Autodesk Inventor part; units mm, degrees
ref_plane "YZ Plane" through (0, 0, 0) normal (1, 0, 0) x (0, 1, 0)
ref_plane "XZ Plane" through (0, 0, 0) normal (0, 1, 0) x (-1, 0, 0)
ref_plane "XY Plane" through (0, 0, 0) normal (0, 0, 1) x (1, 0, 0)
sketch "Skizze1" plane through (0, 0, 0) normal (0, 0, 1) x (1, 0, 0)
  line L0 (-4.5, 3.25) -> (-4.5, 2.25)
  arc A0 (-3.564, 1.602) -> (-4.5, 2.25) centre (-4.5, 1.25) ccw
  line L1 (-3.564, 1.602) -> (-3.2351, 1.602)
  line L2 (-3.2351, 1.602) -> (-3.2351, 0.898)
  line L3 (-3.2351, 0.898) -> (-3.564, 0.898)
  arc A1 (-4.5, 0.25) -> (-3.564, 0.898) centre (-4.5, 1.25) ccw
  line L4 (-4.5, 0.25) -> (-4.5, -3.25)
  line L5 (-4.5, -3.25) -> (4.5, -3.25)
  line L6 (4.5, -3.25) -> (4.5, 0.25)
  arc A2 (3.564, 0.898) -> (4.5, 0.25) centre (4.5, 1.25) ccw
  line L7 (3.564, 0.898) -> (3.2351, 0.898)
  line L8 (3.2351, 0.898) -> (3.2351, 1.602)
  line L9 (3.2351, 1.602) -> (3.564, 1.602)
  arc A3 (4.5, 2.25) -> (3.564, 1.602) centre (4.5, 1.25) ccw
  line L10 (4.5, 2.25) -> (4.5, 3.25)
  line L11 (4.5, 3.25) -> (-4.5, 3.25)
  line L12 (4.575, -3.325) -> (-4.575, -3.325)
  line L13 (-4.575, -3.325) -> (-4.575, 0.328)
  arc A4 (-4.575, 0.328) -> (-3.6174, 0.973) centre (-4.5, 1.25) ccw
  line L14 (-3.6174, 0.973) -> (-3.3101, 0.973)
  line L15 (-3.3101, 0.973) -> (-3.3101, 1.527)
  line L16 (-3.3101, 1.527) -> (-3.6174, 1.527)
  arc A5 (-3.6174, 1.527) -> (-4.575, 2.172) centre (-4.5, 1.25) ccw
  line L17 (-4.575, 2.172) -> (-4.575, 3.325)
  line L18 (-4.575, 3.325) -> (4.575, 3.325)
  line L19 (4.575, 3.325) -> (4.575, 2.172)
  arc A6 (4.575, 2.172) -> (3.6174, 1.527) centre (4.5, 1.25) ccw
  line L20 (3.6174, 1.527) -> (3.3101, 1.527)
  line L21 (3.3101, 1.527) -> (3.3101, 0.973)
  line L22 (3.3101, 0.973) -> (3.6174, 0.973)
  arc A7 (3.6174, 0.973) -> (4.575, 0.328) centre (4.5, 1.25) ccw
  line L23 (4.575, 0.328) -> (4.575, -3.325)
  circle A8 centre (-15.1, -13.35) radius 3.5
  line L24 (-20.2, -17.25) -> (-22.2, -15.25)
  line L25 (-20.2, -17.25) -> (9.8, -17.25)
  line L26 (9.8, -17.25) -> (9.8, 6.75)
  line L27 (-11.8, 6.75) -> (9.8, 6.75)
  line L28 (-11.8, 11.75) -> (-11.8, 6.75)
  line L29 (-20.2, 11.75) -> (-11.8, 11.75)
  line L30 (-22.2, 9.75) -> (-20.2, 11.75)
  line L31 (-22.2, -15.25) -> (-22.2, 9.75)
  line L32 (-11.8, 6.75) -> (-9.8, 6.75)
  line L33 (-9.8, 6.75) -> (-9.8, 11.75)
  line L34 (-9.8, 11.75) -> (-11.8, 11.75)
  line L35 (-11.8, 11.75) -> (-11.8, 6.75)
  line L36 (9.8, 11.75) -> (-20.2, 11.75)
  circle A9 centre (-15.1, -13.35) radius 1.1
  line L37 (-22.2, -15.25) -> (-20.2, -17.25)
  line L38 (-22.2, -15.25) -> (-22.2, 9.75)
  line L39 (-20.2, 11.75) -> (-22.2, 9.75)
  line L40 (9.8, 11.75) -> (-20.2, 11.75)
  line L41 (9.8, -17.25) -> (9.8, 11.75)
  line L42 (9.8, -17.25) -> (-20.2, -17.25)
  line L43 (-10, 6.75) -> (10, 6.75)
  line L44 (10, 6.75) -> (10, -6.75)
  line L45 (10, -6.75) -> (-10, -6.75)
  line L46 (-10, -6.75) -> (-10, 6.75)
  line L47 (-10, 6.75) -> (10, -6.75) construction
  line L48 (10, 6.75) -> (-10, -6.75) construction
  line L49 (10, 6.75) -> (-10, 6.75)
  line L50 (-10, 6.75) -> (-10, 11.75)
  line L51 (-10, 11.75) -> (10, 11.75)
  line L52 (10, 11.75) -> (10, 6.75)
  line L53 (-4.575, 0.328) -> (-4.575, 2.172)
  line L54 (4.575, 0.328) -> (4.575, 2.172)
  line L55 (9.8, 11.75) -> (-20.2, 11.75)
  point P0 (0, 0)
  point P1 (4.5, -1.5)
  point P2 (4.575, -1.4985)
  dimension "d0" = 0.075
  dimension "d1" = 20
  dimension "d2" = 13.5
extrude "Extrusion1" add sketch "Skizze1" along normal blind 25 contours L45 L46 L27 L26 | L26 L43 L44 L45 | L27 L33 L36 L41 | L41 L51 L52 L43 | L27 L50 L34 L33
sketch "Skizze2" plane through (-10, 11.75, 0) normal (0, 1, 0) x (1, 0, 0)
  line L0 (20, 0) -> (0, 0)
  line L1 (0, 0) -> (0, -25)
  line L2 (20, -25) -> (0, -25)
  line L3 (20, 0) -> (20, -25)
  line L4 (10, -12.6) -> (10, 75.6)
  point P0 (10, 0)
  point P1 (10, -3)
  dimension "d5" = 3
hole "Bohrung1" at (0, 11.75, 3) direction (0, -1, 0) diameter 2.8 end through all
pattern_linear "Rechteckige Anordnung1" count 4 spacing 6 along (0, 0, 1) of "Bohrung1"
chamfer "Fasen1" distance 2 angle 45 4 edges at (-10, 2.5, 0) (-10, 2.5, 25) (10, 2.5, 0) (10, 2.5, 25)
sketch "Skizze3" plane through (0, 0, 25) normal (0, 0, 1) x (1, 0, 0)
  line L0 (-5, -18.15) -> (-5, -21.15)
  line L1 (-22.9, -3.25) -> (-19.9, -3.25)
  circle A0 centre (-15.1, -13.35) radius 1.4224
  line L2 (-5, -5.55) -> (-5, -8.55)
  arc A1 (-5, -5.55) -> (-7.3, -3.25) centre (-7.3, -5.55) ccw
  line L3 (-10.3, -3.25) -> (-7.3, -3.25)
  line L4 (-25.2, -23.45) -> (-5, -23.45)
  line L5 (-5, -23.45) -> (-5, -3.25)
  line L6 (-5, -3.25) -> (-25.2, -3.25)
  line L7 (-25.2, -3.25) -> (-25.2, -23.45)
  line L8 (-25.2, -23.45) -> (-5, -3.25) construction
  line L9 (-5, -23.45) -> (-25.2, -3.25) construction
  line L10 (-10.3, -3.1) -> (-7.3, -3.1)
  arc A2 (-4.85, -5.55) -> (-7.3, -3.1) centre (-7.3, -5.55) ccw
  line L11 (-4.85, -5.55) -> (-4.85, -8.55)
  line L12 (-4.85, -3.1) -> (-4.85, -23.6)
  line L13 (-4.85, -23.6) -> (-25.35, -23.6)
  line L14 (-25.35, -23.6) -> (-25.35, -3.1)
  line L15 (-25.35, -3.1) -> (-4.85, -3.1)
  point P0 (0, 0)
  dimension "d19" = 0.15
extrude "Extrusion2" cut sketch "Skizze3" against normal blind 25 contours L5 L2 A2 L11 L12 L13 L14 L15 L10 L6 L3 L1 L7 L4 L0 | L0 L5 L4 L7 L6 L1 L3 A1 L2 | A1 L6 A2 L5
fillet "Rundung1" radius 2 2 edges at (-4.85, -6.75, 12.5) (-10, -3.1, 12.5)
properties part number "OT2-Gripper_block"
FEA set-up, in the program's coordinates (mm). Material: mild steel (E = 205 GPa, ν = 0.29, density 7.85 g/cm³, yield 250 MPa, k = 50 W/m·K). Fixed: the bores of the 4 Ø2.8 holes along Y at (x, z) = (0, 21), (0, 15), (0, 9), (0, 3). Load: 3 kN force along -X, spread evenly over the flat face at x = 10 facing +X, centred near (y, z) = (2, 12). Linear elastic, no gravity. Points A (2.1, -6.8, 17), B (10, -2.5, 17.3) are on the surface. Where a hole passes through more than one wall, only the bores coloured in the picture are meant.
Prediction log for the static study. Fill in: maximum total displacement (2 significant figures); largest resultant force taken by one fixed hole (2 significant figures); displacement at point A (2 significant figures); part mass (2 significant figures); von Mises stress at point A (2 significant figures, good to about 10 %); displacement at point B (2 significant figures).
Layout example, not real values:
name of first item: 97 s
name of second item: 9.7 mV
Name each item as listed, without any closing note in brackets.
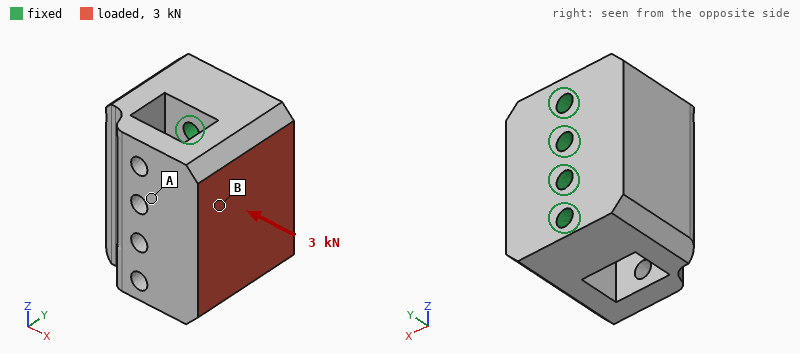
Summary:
maximum total displacement: 5.3 µm
largest resultant force taken by one fixed hole: 820 N
displacement at point A: 4.2 µm
part mass: 54 g
von Mises stress at point A: 23 MPa
displacement at point B: 4.2 µm
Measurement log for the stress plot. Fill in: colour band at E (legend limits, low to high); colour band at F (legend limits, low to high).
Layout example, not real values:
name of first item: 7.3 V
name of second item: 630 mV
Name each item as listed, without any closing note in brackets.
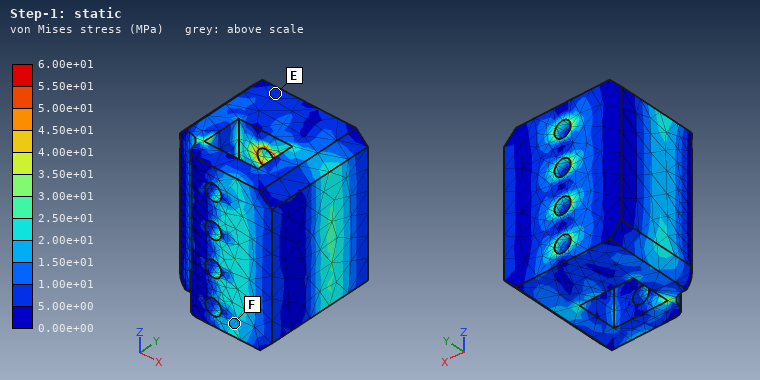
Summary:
colour band at E: 5.00e+00 to 1.00e+01 MPa
colour band at F: 1.50e+01 to 2.00e+01 MPa
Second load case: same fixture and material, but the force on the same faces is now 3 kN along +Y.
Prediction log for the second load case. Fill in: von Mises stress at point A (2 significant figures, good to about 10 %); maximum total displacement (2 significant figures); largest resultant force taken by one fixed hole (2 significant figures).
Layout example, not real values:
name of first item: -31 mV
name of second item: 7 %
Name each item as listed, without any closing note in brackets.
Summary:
von Mises stress at point A: 17 MPa
maximum total displacement: 7.0 µm
largest resultant force taken by one fixed hole: 810 N
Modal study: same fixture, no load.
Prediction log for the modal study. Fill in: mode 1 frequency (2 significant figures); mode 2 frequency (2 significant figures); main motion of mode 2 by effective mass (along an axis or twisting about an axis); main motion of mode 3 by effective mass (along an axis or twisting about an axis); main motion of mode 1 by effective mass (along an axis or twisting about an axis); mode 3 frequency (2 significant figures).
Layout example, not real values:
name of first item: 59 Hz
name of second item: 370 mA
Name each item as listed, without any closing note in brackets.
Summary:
mode 1 frequency: 21 kHz
mode 2 frequency: 29 kHz
main motion of mode 2 by effective mass: along Z
main motion of mode 3 by effective mass: twisting about Y
main motion of mode 1 by effective mass: along X
mode 3 frequency: 38 kHz
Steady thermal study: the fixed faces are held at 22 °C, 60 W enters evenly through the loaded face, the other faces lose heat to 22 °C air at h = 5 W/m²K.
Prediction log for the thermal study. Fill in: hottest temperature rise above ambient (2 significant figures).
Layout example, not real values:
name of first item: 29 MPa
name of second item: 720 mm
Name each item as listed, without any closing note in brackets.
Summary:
hottest temperature rise above ambient: 61 K
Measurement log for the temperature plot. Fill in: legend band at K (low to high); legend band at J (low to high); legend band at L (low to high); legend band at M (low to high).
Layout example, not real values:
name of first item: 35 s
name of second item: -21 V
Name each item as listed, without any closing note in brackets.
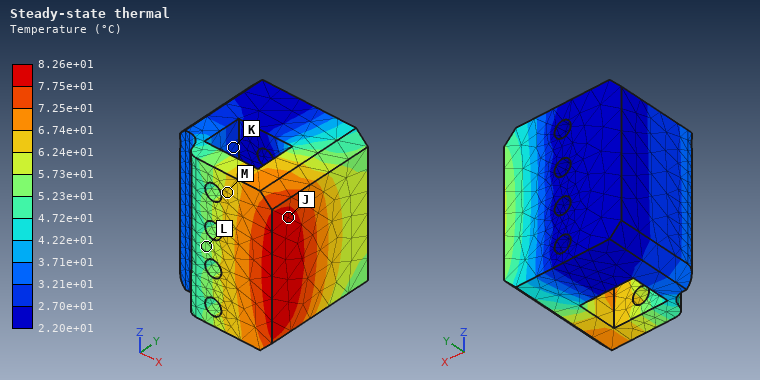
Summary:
legend band at K: 2.70e+01 to 3.21e+01 °C
legend band at J: 7.75e+01 to 8.26e+01 °C
legend band at L: 5.23e+01 to 5.73e+01 °C
legend band at M: 6.24e+01 to 6.74e+01 °C
